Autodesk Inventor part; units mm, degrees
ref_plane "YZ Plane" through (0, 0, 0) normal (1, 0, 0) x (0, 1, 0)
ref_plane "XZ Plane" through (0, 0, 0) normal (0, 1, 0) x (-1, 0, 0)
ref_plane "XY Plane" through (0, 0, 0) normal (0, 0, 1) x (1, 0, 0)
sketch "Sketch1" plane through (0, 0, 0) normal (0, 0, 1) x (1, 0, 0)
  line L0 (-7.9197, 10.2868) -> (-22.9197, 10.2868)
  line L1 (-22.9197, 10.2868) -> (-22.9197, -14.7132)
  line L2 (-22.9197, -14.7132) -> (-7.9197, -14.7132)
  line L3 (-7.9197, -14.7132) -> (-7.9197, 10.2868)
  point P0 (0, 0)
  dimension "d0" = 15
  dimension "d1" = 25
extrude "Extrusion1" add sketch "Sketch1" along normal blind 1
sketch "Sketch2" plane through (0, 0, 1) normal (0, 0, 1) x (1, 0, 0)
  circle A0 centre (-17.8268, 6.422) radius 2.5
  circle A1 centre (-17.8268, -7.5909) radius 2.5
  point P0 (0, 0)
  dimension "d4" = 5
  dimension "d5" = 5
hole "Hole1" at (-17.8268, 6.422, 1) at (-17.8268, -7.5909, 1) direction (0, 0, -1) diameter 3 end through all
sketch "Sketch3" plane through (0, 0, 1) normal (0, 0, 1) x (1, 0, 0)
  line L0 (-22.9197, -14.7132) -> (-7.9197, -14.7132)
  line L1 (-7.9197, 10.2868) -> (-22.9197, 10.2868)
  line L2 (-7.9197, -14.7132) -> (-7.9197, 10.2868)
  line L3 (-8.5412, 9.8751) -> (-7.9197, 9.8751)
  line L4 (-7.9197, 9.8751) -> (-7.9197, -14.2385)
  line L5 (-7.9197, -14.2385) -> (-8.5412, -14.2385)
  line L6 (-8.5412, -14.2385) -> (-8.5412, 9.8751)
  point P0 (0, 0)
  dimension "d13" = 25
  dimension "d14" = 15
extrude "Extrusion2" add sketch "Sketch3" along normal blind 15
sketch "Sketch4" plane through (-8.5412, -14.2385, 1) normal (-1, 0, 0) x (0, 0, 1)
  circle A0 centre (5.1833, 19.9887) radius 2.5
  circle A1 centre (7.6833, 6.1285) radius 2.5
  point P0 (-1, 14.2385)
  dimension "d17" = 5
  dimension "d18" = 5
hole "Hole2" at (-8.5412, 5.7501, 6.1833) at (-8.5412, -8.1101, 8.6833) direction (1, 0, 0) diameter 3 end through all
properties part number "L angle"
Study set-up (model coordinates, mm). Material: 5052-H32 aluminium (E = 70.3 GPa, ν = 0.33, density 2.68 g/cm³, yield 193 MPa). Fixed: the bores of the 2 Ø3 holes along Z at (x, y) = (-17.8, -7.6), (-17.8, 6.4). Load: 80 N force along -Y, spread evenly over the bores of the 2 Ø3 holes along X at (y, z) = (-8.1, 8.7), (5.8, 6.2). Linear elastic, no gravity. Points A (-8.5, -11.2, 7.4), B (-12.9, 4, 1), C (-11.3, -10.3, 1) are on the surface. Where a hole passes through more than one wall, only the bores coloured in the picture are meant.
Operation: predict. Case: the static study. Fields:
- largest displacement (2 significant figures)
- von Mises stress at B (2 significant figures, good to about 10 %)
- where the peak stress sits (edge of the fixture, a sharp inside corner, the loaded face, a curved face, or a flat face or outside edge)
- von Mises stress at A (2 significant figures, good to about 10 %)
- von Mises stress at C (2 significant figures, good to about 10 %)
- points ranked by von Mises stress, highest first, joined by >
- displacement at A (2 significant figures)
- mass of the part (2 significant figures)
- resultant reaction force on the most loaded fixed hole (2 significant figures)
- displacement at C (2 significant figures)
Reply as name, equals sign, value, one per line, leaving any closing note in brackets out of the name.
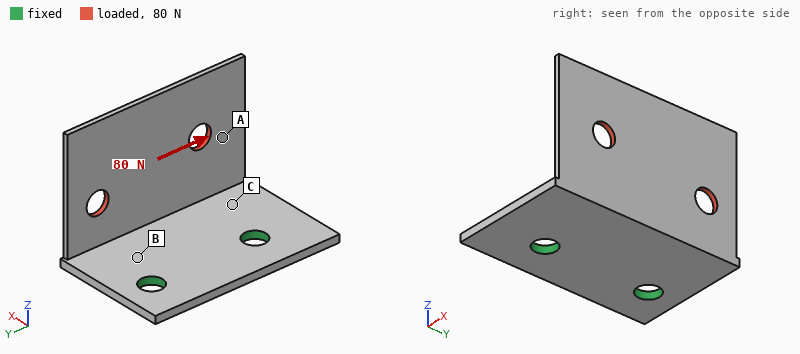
largest displacement = 0.20 mm
von Mises stress at B = 70 MPa
where the peak stress sits = a flat face or outside edge
von Mises stress at A = 22 MPa
von Mises stress at C = 42 MPa
points ranked by von Mises stress, highest first, joined by > = B > C > A
displacement at A = 0.12 mm
mass of the part = 1.5 g
resultant reaction force on the most loaded fixed hole = 70 N
displacement at C = 0.044 mm
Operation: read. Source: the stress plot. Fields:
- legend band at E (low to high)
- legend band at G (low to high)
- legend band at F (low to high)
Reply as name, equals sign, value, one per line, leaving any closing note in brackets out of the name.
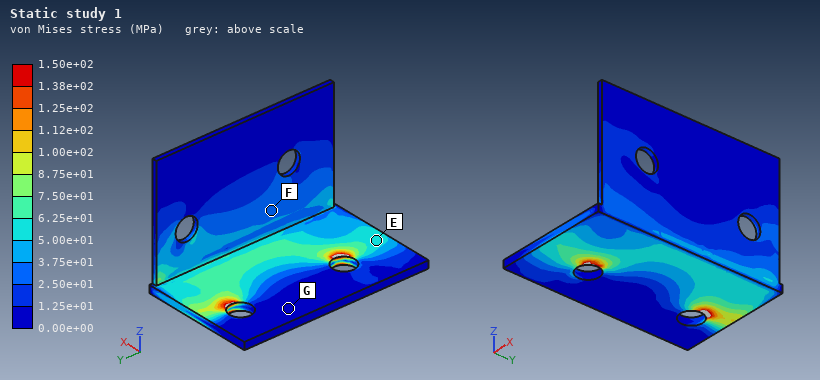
legend band at E = 5.00e+01 to 6.25e+01 MPa
legend band at G = 0.00e+00 to 1.25e+01 MPa
legend band at F = 2.50e+01 to 3.75e+01 MPa
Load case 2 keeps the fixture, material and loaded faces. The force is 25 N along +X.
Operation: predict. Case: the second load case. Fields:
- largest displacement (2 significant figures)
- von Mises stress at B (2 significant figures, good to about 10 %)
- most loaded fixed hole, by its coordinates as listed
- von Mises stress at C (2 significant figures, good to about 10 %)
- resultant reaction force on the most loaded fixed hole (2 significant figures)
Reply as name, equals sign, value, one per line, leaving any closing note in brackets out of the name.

largest displacement = 0.37 mm
von Mises stress at B = 38 MPa
most loaded fixed hole, by its coordinates as listed = (-17.8, -7.6)
von Mises stress at C = 38 MPa
resultant reaction force on the most loaded fixed hole = 14 N
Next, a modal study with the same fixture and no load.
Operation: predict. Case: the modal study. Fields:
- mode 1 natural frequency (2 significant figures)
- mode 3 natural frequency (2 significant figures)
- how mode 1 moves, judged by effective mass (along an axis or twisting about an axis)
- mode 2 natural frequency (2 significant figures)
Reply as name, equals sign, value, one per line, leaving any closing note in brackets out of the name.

mode 1 natural frequency = 1800 Hz
mode 3 natural frequency = 4800 Hz
how mode 1 moves, judged by effective mass = along X
mode 2 natural frequency = 3400 Hz
